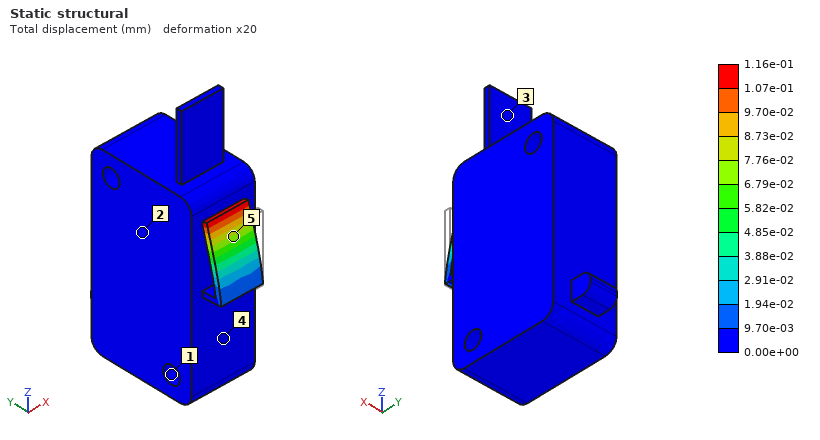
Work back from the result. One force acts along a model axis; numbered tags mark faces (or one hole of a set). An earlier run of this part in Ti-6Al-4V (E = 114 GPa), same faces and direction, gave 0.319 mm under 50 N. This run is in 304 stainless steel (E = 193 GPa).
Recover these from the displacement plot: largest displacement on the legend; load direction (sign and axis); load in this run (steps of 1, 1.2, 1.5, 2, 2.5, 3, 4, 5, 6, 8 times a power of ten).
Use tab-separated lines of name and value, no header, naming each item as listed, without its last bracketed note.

largest displacement on the legend	1.16e-01 mm
load direction	+Y
load in this run	30 N
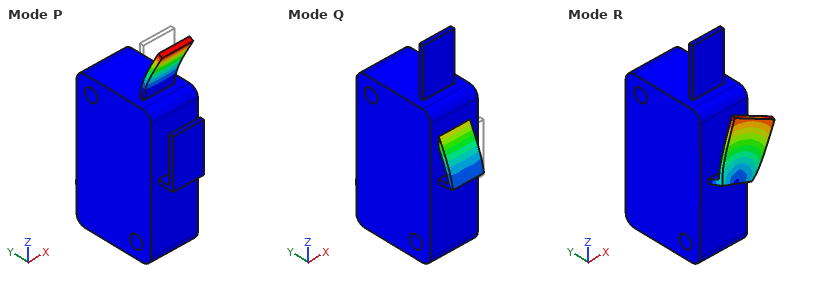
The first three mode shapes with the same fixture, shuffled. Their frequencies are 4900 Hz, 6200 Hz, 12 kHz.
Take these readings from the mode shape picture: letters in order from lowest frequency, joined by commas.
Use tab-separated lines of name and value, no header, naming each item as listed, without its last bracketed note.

letters in order from lowest frequency, joined by commas	Q, P, R
